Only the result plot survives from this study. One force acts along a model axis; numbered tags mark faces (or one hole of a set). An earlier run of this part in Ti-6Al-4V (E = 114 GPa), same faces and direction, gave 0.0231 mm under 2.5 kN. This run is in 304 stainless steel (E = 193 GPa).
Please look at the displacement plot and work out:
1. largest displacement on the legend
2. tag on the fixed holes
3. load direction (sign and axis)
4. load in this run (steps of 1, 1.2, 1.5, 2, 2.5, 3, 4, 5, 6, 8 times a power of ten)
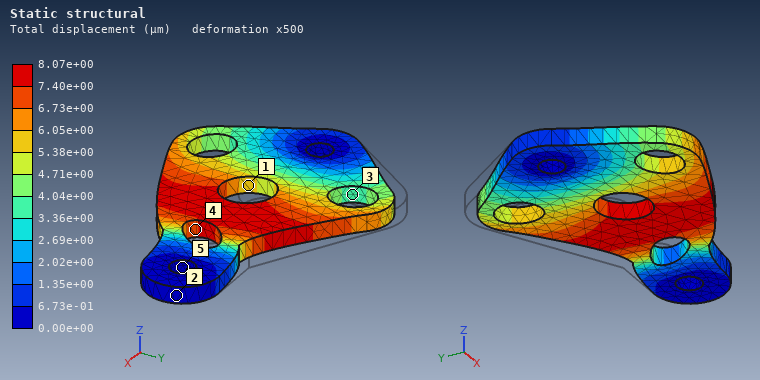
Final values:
8.07e+00 µm
5
-Y
1.5 kN
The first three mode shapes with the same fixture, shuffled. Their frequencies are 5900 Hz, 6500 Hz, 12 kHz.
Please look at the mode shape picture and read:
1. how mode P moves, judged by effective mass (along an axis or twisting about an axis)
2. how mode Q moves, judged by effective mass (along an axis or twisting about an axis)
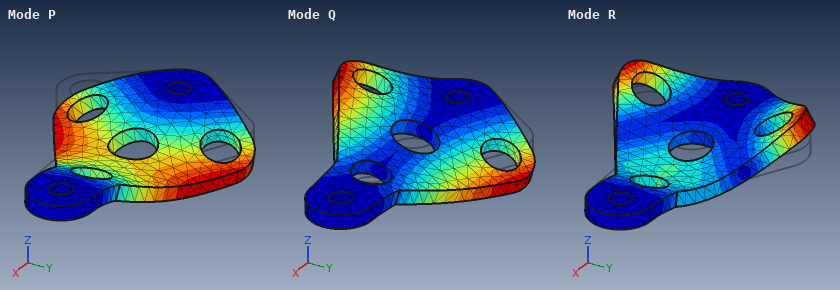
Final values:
along Z
twisting about X
